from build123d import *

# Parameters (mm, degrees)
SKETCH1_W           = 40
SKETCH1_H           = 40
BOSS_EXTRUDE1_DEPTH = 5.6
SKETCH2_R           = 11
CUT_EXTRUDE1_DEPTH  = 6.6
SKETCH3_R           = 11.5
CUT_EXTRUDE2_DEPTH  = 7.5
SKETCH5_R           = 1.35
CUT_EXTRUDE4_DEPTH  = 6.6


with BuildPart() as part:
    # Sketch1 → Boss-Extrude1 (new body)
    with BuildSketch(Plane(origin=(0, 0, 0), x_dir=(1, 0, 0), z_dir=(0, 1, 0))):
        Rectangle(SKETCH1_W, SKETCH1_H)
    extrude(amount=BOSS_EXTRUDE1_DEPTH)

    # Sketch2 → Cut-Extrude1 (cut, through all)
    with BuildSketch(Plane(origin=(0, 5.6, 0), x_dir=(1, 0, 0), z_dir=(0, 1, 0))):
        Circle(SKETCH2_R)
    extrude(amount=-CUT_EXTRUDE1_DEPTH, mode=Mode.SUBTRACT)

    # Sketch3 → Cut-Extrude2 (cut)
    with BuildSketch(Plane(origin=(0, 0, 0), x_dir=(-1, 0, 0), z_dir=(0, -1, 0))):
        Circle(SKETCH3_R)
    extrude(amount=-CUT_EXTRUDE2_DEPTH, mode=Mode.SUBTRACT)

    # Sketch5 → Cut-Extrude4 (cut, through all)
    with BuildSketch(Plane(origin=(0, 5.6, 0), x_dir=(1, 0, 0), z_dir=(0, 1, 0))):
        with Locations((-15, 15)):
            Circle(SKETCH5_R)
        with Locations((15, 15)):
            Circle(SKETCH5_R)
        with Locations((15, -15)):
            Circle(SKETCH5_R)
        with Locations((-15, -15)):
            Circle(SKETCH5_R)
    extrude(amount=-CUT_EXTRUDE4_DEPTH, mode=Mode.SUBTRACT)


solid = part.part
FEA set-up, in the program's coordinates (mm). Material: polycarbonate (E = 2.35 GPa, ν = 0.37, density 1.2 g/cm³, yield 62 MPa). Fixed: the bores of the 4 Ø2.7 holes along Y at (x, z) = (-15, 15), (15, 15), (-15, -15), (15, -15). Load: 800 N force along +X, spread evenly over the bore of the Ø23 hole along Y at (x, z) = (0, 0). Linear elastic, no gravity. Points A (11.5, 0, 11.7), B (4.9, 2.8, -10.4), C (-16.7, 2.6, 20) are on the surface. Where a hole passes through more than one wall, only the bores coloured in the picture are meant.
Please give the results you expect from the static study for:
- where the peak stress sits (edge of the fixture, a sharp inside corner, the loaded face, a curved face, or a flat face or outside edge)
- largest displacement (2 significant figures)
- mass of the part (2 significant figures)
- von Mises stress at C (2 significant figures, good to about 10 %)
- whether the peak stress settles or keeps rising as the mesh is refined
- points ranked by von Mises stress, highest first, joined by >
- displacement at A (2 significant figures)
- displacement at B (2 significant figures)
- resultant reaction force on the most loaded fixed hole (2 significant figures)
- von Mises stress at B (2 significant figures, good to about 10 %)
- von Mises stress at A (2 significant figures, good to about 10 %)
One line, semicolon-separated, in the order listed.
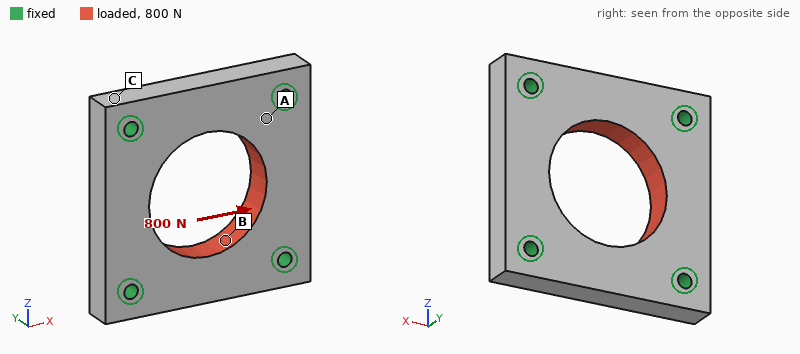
edge of the fixture; 46 µm; 7.8 g; 1.4 MPa; keeps rising; B > A > C; 13 µm; 20 µm; 200 N; 4.6 MPa; 3.4 MPa
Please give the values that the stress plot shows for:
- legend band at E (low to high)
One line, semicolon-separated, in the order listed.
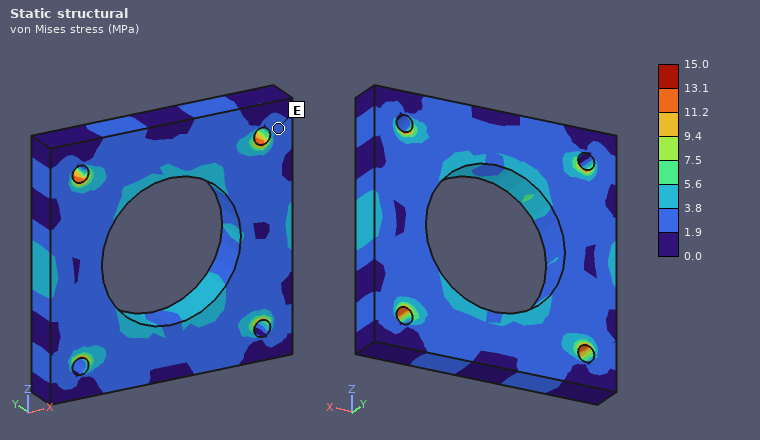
1.9 to 3.8 MPa
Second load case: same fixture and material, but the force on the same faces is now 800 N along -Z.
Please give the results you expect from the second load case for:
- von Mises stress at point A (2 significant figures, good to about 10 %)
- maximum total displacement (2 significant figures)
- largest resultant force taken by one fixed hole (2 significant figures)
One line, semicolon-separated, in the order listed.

3.4 MPa; 46 µm; 200 N
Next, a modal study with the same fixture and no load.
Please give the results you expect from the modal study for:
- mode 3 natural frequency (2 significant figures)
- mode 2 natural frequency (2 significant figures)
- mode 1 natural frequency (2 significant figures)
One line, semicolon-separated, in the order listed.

7500 Hz; 7200 Hz; 7100 Hz
